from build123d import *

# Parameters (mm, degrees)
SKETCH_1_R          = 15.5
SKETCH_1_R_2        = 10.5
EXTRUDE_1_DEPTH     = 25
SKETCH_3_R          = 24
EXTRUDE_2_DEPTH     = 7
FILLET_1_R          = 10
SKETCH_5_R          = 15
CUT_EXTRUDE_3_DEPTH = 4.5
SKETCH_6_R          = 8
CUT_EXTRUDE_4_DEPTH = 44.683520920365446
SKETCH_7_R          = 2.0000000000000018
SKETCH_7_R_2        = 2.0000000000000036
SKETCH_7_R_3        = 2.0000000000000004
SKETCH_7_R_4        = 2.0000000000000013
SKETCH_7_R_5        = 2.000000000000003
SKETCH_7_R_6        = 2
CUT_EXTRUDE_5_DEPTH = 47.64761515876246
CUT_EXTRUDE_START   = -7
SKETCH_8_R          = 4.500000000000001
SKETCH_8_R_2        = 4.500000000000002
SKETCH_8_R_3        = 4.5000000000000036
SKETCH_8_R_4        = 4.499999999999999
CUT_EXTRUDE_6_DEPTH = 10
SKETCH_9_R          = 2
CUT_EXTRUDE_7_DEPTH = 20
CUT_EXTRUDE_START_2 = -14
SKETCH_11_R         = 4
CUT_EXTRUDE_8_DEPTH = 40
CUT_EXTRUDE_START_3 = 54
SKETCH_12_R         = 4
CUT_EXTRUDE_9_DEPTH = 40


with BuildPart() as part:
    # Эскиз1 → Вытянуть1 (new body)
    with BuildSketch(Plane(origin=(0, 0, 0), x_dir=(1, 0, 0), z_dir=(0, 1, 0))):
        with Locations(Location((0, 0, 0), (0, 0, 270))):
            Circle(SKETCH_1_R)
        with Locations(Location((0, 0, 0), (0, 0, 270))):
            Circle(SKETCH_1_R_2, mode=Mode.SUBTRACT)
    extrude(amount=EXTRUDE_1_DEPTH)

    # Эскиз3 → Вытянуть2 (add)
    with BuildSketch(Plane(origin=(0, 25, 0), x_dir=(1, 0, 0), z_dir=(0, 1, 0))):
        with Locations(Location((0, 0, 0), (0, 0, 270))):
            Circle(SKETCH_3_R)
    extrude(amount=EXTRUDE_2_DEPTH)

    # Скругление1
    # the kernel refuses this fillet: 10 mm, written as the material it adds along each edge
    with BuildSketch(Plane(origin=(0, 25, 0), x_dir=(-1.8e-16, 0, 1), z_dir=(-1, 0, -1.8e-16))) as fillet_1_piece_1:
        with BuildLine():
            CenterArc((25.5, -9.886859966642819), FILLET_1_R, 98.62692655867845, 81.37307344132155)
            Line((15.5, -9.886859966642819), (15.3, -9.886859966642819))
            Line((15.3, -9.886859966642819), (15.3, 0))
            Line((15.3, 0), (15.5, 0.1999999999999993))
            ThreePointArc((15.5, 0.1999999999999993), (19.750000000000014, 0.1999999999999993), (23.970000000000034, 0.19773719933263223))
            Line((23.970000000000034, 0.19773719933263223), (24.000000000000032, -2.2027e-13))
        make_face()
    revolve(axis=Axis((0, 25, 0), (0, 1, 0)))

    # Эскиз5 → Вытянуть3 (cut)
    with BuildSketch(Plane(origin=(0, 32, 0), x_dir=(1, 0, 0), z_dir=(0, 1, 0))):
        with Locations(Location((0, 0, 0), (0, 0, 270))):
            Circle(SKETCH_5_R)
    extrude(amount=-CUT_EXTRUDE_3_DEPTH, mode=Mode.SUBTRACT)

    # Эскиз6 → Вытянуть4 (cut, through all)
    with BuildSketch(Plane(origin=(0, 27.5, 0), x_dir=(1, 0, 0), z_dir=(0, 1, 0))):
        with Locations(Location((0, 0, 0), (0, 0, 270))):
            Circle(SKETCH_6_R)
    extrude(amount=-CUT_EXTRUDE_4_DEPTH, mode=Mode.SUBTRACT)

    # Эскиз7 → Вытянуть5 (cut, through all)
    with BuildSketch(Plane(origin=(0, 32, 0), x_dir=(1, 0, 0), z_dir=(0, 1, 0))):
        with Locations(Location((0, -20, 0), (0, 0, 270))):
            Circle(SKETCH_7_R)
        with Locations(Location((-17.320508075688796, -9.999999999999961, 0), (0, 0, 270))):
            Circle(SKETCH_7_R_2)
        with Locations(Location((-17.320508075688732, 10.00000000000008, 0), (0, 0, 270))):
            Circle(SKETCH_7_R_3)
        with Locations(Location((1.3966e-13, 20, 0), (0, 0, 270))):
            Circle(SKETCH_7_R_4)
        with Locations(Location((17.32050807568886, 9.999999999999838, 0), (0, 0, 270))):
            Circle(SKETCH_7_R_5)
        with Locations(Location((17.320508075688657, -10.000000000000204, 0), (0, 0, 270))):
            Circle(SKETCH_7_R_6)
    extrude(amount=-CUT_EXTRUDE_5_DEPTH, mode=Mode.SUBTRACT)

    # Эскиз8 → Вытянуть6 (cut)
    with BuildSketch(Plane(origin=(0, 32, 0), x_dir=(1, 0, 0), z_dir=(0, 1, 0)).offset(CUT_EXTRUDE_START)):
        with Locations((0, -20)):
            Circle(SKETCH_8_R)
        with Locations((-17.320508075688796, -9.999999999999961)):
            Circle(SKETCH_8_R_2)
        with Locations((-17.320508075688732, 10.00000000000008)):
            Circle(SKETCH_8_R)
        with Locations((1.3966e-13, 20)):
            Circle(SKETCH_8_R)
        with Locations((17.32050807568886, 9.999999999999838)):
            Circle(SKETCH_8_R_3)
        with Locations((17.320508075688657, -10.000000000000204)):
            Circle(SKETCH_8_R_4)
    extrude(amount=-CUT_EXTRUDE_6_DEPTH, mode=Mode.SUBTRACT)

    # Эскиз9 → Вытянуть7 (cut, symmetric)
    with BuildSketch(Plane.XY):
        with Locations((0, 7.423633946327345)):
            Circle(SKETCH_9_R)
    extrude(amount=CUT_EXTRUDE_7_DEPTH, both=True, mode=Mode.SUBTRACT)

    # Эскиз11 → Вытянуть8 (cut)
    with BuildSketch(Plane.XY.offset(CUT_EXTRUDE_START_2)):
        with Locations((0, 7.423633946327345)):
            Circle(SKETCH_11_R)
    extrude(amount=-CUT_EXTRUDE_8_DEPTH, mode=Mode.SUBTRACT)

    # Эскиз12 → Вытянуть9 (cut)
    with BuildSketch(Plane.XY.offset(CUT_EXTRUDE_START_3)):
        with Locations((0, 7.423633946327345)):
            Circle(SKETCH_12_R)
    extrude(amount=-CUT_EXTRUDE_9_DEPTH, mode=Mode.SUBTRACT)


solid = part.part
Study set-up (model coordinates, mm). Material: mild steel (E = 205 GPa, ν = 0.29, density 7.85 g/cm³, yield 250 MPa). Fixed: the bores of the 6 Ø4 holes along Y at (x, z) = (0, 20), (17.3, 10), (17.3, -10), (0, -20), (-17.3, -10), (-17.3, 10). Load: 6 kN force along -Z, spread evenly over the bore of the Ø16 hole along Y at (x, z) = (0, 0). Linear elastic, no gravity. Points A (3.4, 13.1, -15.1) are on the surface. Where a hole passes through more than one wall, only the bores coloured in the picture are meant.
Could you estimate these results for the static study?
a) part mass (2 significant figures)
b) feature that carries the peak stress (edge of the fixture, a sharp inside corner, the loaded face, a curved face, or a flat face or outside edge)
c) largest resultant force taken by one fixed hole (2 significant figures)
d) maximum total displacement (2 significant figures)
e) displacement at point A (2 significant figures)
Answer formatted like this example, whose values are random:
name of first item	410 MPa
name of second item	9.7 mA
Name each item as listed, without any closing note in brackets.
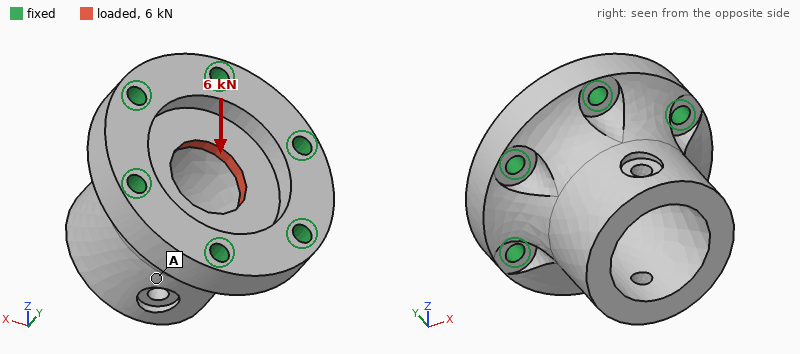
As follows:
part mass	160 g
feature that carries the peak stress	a sharp inside corner
largest resultant force taken by one fixed hole	1.3 kN
maximum total displacement	2.5 µm
displacement at point A	0.69 µm
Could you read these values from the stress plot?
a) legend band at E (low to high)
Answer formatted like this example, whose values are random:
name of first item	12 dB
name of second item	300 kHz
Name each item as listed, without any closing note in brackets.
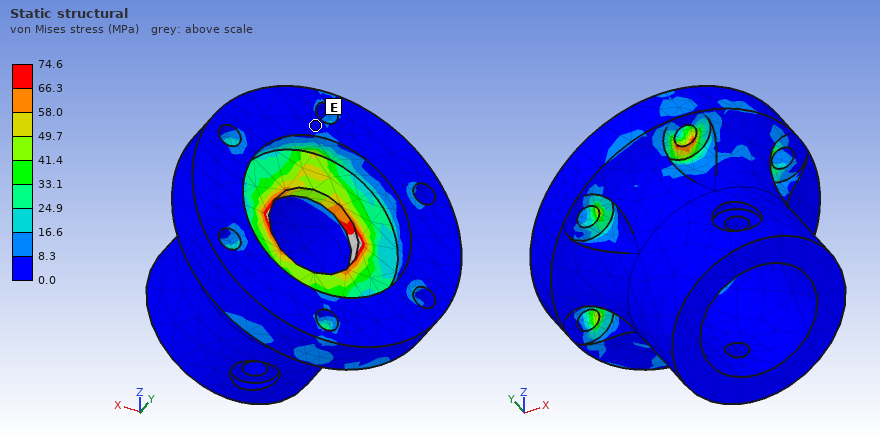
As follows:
legend band at E	0.0 to 8.3 MPa
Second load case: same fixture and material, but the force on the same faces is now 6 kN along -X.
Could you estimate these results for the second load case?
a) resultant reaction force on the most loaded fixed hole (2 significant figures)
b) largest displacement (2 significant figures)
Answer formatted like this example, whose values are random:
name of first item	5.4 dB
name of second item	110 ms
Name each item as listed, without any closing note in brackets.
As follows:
resultant reaction force on the most loaded fixed hole	1.2 kN
largest displacement	2.6 µm
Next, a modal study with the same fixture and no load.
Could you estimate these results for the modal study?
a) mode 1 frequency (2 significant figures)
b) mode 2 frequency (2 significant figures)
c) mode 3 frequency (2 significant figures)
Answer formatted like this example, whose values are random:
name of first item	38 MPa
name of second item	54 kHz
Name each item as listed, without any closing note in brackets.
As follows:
mode 1 frequency	19 kHz
mode 2 frequency	19 kHz
mode 3 frequency	23 kHz
